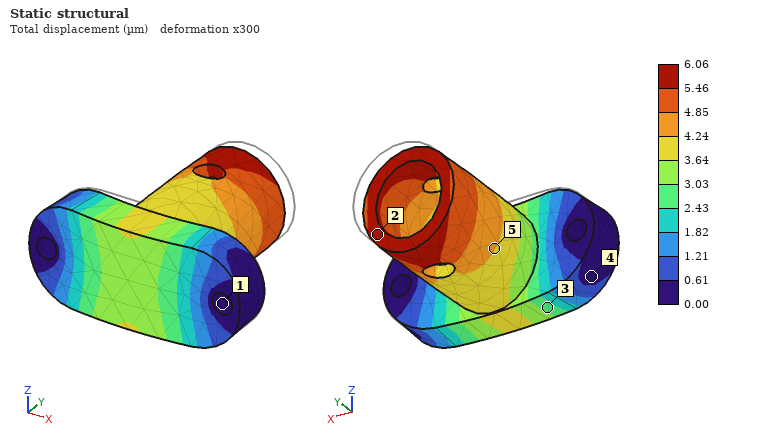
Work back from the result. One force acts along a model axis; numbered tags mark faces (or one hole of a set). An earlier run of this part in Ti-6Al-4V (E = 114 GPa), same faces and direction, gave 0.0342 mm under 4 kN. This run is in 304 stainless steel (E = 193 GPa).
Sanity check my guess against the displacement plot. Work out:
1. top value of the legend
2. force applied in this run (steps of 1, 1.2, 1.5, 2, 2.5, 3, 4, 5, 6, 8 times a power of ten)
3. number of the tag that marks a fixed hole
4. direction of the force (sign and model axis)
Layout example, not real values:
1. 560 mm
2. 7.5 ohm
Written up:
1. 6.06 µm
2. 1.2 kN
3. 1
4. -Y
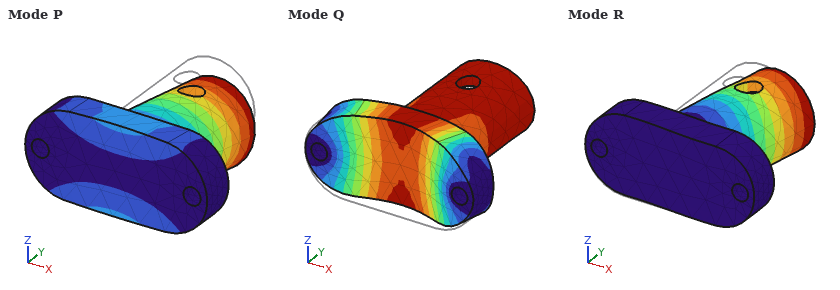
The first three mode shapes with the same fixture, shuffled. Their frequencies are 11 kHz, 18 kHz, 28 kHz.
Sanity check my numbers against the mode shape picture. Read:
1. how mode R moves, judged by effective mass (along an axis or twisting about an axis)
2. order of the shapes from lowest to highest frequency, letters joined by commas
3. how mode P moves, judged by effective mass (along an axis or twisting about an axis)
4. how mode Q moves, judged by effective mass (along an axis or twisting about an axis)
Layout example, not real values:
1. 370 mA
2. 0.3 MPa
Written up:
1. along X
2. P, R, Q
3. along Z
4. along Y
